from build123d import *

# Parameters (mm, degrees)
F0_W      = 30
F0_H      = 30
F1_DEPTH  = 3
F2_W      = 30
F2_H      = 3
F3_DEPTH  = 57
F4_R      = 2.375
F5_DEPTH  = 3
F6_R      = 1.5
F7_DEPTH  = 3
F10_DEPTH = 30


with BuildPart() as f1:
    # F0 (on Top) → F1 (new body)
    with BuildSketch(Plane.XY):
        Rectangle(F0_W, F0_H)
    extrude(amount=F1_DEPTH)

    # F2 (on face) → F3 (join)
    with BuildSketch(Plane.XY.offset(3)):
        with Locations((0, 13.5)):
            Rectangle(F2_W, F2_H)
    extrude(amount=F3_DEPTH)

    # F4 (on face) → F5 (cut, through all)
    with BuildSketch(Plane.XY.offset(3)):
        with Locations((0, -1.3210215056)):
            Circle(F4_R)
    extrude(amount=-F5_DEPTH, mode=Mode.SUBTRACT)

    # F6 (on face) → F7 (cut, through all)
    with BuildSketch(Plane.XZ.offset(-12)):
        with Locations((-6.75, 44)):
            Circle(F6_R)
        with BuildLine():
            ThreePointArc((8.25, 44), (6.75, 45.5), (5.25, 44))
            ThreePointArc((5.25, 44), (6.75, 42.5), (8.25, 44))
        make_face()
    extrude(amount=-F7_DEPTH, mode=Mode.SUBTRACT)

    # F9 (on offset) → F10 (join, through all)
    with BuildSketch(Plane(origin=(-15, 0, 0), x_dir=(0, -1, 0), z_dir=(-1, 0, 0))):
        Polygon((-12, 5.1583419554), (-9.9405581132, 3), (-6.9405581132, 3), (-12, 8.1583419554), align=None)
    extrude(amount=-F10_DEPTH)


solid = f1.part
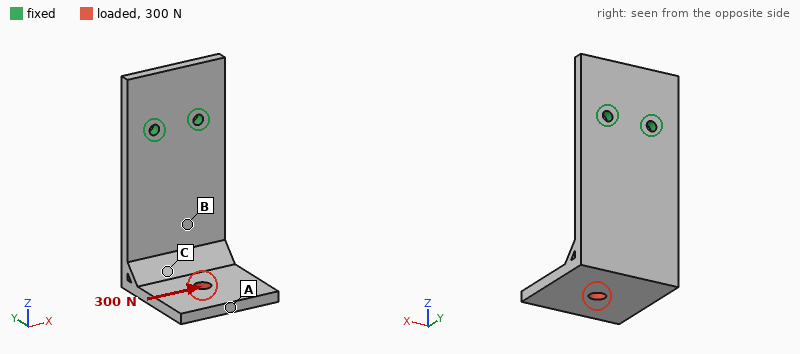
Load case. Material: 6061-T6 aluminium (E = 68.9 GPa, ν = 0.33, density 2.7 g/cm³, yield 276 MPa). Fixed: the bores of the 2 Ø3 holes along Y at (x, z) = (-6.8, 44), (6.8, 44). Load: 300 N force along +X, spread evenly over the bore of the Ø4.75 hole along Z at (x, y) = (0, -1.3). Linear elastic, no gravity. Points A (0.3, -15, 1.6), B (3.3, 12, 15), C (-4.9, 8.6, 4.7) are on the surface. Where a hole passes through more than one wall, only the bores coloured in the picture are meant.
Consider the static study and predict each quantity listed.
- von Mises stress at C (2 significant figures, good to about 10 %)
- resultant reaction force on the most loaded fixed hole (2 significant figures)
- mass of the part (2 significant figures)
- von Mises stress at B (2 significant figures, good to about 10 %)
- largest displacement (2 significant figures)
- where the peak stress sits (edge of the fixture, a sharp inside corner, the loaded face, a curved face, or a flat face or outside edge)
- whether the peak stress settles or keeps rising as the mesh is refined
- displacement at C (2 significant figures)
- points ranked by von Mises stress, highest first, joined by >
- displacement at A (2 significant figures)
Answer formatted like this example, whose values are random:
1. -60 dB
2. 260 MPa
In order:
1. 38 MPa
2. 880 N
3. 22 g
4. 75 MPa
5. 0.62 mm
6. edge of the fixture
7. keeps rising
8. 0.15 mm
9. B > C > A
10. 0.55 mm
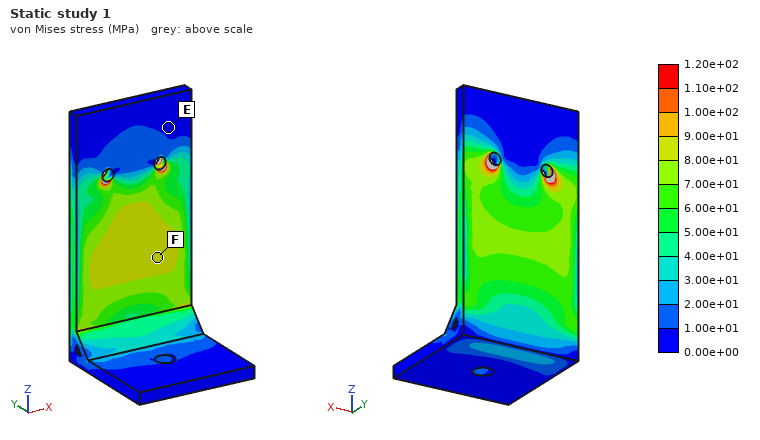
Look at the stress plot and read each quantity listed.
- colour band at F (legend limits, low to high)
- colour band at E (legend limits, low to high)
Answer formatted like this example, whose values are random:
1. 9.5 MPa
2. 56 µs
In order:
1. 8.00e+01 to 9.00e+01 MPa
2. 0.00e+00 to 1.00e+01 MPa
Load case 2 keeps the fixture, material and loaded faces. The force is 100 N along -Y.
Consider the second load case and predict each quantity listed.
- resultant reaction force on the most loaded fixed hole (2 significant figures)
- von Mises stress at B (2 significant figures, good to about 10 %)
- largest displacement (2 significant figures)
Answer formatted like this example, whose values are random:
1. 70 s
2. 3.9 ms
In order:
1. 50 N
2. 28 MPa
3. 0.77 mm
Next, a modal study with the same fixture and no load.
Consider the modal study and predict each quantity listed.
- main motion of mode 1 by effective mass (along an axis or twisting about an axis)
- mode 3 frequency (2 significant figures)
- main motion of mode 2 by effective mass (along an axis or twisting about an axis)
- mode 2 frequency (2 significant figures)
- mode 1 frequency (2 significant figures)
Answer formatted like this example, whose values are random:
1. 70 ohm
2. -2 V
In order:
1. along Y
2. 2600 Hz
3. along X
4. 1500 Hz
5. 620 Hz
